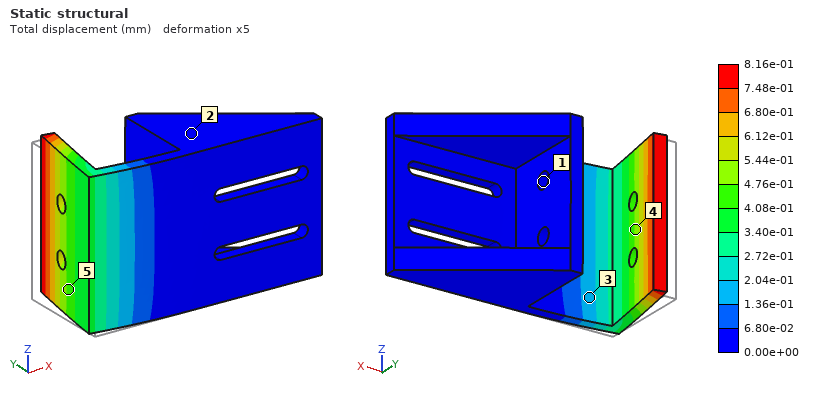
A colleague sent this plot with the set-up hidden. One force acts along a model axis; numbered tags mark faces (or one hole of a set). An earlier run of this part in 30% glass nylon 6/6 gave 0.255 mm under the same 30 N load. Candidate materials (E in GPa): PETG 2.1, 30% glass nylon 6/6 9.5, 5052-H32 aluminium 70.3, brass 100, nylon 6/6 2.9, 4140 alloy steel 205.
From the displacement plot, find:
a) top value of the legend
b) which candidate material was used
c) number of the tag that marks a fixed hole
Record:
8.16e-01 mm
nylon 6/6
1
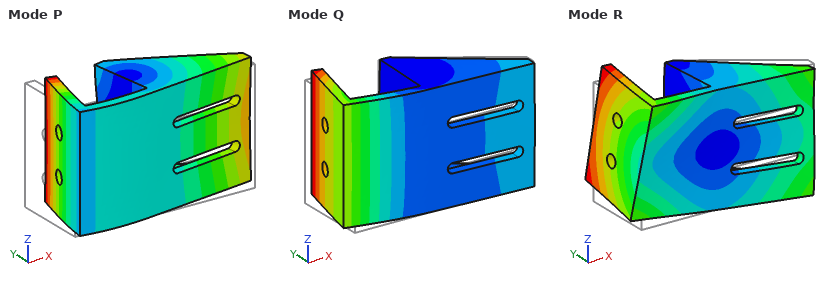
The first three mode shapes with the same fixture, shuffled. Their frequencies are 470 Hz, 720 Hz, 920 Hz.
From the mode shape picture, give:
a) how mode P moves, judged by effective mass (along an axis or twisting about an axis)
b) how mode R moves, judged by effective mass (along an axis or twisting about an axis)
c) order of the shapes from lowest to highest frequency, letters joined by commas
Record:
along X
twisting about Y
Q, R, P
